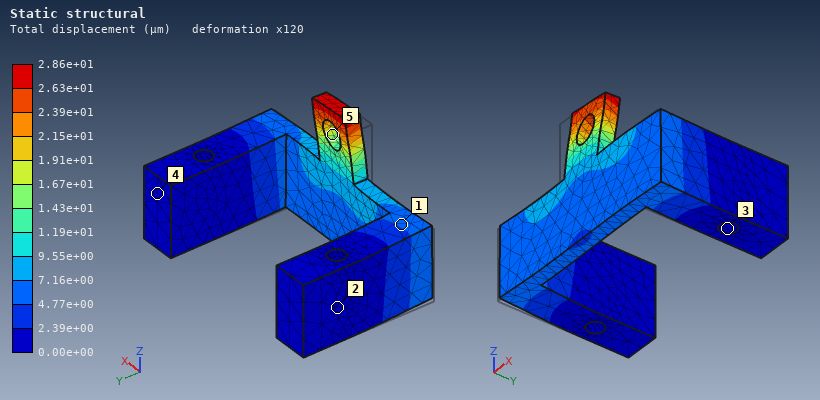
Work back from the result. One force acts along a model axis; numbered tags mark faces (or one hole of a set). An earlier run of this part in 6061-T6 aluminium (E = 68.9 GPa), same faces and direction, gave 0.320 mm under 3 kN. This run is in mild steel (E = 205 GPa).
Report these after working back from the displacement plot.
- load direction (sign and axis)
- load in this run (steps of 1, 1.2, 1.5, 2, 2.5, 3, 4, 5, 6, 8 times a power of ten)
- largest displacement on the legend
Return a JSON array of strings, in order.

["+X", "800 N", "2.86e+01 µm"]
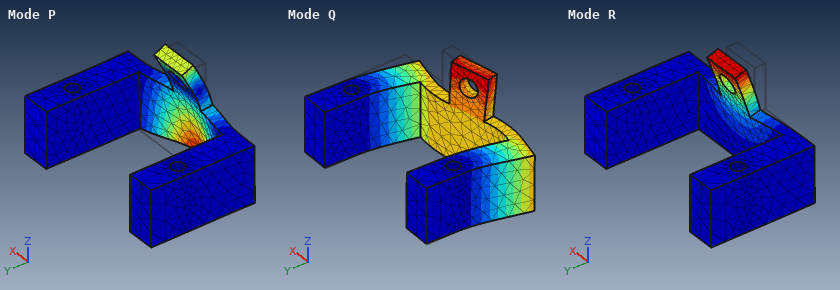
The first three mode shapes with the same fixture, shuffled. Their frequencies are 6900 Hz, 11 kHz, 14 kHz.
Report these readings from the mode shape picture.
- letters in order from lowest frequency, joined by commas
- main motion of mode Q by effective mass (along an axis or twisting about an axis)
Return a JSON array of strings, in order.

["R, Q, P", "along X"]
